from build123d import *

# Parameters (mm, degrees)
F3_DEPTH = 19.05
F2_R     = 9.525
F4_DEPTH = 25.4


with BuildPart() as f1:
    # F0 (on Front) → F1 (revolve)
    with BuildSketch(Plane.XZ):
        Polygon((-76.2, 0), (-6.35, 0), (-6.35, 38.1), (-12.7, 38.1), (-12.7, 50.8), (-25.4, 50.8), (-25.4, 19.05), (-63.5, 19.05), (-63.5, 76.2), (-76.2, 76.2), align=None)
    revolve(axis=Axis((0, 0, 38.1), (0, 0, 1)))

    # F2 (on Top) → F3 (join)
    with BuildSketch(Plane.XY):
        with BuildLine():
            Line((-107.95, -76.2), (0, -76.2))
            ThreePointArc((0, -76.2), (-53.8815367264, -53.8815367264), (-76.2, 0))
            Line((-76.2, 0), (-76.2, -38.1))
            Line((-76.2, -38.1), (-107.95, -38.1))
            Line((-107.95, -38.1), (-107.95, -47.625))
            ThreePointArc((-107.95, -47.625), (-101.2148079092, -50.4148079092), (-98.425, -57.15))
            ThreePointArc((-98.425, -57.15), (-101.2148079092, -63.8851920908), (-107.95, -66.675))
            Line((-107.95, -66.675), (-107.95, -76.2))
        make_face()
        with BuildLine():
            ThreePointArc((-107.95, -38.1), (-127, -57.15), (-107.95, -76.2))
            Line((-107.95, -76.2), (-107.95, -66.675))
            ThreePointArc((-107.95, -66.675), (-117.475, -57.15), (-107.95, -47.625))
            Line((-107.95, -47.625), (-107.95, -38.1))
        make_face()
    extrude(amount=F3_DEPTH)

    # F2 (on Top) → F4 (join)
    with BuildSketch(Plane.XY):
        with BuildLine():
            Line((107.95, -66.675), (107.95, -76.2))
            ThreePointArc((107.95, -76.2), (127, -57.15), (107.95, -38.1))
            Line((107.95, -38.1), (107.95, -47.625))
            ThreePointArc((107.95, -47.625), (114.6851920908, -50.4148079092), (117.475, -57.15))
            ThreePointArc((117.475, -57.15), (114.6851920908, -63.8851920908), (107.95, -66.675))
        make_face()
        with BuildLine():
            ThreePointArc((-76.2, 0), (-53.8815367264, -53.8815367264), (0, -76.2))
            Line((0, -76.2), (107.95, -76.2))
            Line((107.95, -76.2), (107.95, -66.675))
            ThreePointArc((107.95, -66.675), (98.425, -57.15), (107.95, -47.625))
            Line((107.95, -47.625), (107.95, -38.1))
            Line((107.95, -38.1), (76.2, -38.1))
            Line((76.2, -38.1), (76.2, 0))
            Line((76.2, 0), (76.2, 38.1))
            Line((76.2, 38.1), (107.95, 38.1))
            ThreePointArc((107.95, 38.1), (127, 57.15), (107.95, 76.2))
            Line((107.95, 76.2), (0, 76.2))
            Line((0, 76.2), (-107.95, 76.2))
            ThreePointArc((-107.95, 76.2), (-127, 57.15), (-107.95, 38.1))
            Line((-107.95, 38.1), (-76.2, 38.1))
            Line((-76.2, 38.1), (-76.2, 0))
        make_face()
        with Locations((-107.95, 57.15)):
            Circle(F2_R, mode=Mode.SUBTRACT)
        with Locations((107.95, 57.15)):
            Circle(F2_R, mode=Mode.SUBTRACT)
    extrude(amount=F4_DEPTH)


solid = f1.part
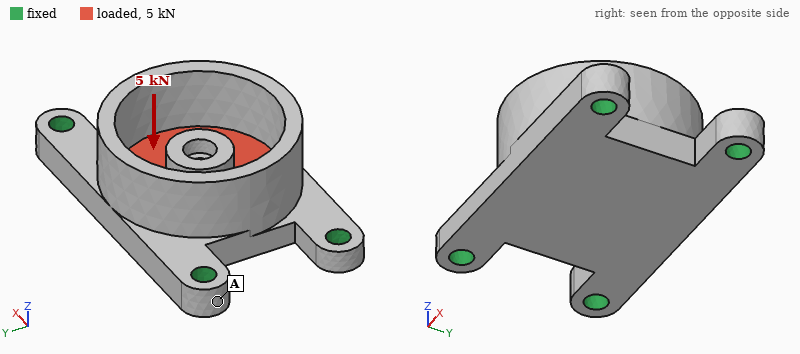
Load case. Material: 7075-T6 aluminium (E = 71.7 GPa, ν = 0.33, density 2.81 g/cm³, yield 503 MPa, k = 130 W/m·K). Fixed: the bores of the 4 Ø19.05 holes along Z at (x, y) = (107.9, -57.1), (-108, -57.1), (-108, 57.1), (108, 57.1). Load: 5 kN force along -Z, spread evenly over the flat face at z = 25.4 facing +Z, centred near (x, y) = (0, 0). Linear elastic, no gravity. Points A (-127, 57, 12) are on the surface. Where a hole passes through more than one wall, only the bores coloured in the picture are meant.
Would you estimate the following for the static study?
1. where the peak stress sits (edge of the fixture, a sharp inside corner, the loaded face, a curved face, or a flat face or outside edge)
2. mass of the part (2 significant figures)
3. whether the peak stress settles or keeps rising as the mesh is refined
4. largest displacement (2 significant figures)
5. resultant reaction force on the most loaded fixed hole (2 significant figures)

edge of the fixture
3.0 kg
keeps rising
17 µm
1.4 kN
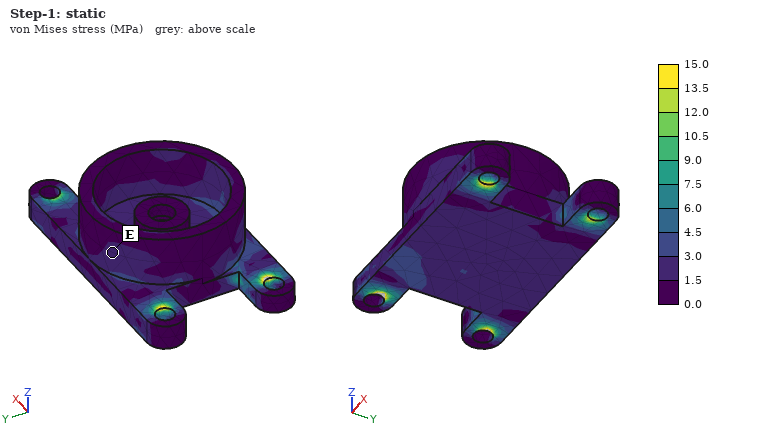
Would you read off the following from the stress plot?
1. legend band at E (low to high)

1.5 to 3.0 MPa
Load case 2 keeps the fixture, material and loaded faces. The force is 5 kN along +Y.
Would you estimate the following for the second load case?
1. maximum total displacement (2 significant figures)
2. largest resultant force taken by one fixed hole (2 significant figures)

8.1 µm
1.6 kN
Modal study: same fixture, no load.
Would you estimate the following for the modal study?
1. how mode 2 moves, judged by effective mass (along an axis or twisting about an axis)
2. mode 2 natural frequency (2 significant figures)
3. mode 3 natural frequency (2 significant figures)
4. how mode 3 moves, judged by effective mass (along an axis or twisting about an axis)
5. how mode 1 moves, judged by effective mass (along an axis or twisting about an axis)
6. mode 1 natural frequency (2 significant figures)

along Y
2500 Hz
3600 Hz
along Y
along Z
2100 Hz
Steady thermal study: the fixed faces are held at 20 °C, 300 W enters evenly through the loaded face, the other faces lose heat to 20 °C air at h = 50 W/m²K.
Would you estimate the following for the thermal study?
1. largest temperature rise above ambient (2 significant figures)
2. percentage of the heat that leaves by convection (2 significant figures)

28 K
34 %
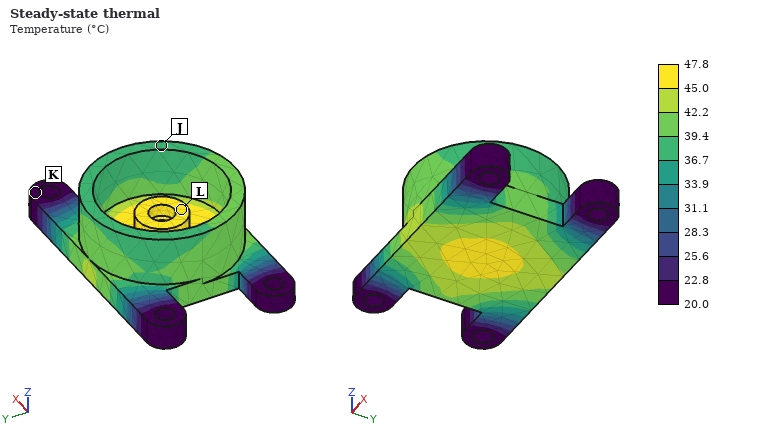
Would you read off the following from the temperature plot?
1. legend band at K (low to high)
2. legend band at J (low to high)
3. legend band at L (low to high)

20.0 to 22.8 °C
36.7 to 39.4 °C
45.0 to 47.8 °C
